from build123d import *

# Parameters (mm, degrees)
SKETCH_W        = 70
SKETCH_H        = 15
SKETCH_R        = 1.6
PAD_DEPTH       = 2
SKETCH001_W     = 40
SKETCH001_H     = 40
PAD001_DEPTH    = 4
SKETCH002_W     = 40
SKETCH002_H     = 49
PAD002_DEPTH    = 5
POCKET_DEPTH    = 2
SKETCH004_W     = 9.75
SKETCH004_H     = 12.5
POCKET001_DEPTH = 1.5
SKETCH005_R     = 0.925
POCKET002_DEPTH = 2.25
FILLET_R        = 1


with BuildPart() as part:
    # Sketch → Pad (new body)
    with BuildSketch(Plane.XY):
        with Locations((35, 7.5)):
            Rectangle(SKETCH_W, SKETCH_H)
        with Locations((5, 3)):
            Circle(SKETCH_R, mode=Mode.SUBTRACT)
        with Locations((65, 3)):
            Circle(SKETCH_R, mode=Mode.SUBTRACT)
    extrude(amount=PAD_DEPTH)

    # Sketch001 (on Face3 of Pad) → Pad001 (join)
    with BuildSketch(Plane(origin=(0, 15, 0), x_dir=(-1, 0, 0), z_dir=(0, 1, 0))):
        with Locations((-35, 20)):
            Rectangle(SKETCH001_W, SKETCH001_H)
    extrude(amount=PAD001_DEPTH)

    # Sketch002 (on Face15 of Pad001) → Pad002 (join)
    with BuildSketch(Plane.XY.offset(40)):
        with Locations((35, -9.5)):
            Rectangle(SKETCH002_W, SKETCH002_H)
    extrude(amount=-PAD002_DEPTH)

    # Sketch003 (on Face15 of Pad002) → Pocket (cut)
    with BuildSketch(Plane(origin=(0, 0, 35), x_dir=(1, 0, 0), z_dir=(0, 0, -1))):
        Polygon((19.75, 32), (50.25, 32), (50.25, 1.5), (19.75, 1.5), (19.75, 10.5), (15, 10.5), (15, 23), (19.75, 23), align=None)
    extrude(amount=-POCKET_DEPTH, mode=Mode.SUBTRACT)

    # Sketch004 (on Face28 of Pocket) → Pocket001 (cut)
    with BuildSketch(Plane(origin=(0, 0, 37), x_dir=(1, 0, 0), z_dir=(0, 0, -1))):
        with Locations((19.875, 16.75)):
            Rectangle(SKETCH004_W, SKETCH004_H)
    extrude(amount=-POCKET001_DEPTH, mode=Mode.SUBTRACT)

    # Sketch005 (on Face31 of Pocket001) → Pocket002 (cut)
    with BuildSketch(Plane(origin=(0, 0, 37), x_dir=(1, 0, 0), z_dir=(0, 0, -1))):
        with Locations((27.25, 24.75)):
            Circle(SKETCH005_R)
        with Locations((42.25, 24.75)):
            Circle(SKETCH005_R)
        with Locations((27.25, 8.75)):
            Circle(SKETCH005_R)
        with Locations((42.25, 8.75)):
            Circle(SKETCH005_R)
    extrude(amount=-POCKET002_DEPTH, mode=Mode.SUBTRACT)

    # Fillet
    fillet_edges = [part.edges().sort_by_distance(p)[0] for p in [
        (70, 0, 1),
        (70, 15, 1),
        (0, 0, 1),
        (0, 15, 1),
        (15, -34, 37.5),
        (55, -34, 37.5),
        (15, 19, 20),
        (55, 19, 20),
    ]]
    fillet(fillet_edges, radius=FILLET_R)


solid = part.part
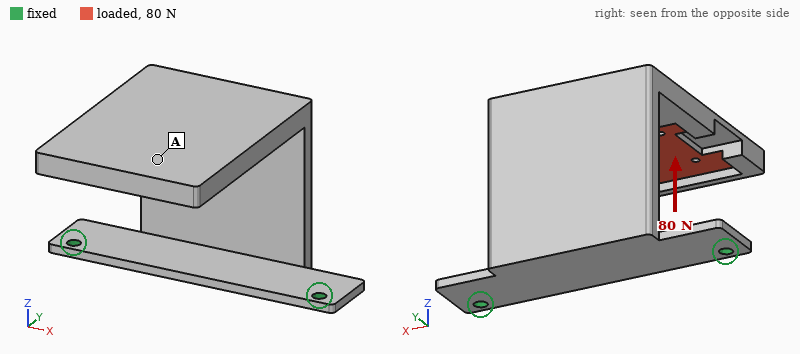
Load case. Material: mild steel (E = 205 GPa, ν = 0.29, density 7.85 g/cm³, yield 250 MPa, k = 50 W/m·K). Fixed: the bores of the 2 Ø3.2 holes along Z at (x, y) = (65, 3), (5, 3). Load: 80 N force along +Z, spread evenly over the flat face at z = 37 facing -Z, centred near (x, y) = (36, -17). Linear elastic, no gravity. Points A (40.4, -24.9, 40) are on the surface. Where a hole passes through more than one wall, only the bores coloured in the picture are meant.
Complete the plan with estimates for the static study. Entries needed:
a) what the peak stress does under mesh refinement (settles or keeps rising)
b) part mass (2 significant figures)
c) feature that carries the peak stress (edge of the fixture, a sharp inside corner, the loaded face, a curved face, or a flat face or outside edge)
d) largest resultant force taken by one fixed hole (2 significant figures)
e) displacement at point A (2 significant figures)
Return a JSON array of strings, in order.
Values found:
["keeps rising", "130 g", "edge of the fixture", "42 N", "0.48 mm"]
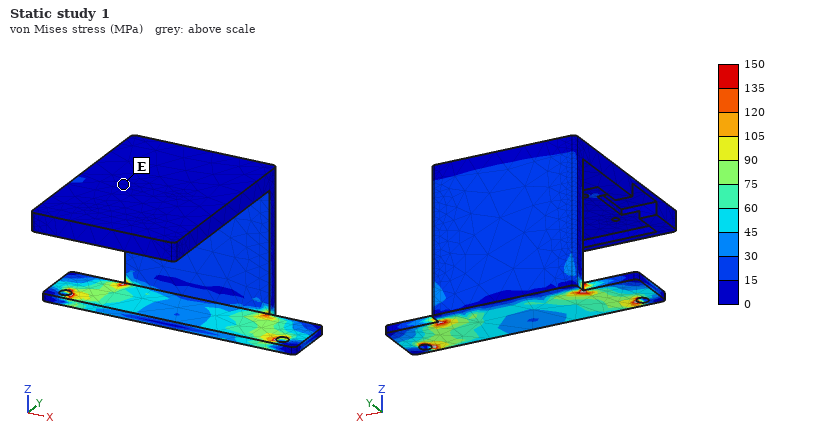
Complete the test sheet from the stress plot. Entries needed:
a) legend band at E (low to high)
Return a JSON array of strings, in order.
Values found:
["0 to 15 MPa"]
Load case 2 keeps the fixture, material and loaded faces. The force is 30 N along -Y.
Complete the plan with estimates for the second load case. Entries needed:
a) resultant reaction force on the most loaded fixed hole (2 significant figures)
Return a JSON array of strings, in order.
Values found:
["22 N"]
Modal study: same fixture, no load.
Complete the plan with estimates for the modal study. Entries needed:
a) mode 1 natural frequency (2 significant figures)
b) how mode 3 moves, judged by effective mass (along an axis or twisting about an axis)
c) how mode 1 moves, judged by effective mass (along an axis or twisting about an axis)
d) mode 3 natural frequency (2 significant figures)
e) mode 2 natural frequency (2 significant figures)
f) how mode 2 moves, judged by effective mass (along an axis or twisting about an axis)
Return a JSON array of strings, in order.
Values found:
["220 Hz", "along Z", "along Y", "920 Hz", "650 Hz", "along X"]
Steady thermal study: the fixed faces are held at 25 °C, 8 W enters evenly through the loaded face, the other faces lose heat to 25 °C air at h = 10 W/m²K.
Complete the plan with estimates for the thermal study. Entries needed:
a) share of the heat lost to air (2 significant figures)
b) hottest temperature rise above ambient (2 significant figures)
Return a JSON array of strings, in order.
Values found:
["53 %", "75 K"]
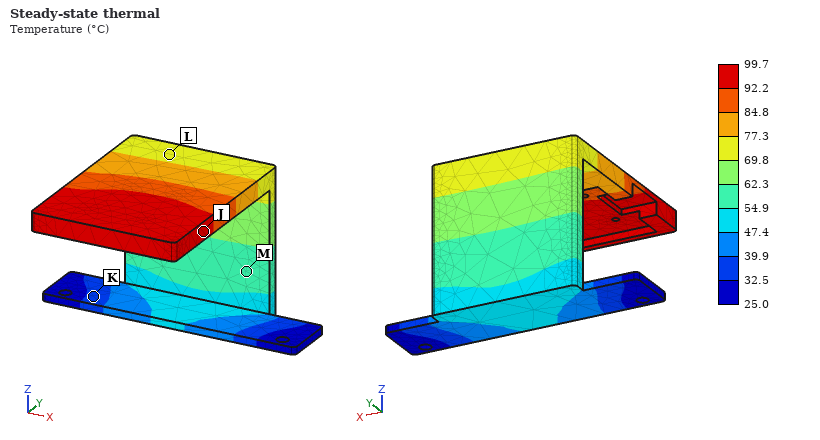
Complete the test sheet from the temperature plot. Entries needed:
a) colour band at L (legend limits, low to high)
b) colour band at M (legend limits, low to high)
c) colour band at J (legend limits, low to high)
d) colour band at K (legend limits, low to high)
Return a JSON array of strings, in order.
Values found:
["69.8 to 77.3 °C", "54.9 to 62.3 °C", "92.2 to 99.7 °C", "32.5 to 39.9 °C"]
